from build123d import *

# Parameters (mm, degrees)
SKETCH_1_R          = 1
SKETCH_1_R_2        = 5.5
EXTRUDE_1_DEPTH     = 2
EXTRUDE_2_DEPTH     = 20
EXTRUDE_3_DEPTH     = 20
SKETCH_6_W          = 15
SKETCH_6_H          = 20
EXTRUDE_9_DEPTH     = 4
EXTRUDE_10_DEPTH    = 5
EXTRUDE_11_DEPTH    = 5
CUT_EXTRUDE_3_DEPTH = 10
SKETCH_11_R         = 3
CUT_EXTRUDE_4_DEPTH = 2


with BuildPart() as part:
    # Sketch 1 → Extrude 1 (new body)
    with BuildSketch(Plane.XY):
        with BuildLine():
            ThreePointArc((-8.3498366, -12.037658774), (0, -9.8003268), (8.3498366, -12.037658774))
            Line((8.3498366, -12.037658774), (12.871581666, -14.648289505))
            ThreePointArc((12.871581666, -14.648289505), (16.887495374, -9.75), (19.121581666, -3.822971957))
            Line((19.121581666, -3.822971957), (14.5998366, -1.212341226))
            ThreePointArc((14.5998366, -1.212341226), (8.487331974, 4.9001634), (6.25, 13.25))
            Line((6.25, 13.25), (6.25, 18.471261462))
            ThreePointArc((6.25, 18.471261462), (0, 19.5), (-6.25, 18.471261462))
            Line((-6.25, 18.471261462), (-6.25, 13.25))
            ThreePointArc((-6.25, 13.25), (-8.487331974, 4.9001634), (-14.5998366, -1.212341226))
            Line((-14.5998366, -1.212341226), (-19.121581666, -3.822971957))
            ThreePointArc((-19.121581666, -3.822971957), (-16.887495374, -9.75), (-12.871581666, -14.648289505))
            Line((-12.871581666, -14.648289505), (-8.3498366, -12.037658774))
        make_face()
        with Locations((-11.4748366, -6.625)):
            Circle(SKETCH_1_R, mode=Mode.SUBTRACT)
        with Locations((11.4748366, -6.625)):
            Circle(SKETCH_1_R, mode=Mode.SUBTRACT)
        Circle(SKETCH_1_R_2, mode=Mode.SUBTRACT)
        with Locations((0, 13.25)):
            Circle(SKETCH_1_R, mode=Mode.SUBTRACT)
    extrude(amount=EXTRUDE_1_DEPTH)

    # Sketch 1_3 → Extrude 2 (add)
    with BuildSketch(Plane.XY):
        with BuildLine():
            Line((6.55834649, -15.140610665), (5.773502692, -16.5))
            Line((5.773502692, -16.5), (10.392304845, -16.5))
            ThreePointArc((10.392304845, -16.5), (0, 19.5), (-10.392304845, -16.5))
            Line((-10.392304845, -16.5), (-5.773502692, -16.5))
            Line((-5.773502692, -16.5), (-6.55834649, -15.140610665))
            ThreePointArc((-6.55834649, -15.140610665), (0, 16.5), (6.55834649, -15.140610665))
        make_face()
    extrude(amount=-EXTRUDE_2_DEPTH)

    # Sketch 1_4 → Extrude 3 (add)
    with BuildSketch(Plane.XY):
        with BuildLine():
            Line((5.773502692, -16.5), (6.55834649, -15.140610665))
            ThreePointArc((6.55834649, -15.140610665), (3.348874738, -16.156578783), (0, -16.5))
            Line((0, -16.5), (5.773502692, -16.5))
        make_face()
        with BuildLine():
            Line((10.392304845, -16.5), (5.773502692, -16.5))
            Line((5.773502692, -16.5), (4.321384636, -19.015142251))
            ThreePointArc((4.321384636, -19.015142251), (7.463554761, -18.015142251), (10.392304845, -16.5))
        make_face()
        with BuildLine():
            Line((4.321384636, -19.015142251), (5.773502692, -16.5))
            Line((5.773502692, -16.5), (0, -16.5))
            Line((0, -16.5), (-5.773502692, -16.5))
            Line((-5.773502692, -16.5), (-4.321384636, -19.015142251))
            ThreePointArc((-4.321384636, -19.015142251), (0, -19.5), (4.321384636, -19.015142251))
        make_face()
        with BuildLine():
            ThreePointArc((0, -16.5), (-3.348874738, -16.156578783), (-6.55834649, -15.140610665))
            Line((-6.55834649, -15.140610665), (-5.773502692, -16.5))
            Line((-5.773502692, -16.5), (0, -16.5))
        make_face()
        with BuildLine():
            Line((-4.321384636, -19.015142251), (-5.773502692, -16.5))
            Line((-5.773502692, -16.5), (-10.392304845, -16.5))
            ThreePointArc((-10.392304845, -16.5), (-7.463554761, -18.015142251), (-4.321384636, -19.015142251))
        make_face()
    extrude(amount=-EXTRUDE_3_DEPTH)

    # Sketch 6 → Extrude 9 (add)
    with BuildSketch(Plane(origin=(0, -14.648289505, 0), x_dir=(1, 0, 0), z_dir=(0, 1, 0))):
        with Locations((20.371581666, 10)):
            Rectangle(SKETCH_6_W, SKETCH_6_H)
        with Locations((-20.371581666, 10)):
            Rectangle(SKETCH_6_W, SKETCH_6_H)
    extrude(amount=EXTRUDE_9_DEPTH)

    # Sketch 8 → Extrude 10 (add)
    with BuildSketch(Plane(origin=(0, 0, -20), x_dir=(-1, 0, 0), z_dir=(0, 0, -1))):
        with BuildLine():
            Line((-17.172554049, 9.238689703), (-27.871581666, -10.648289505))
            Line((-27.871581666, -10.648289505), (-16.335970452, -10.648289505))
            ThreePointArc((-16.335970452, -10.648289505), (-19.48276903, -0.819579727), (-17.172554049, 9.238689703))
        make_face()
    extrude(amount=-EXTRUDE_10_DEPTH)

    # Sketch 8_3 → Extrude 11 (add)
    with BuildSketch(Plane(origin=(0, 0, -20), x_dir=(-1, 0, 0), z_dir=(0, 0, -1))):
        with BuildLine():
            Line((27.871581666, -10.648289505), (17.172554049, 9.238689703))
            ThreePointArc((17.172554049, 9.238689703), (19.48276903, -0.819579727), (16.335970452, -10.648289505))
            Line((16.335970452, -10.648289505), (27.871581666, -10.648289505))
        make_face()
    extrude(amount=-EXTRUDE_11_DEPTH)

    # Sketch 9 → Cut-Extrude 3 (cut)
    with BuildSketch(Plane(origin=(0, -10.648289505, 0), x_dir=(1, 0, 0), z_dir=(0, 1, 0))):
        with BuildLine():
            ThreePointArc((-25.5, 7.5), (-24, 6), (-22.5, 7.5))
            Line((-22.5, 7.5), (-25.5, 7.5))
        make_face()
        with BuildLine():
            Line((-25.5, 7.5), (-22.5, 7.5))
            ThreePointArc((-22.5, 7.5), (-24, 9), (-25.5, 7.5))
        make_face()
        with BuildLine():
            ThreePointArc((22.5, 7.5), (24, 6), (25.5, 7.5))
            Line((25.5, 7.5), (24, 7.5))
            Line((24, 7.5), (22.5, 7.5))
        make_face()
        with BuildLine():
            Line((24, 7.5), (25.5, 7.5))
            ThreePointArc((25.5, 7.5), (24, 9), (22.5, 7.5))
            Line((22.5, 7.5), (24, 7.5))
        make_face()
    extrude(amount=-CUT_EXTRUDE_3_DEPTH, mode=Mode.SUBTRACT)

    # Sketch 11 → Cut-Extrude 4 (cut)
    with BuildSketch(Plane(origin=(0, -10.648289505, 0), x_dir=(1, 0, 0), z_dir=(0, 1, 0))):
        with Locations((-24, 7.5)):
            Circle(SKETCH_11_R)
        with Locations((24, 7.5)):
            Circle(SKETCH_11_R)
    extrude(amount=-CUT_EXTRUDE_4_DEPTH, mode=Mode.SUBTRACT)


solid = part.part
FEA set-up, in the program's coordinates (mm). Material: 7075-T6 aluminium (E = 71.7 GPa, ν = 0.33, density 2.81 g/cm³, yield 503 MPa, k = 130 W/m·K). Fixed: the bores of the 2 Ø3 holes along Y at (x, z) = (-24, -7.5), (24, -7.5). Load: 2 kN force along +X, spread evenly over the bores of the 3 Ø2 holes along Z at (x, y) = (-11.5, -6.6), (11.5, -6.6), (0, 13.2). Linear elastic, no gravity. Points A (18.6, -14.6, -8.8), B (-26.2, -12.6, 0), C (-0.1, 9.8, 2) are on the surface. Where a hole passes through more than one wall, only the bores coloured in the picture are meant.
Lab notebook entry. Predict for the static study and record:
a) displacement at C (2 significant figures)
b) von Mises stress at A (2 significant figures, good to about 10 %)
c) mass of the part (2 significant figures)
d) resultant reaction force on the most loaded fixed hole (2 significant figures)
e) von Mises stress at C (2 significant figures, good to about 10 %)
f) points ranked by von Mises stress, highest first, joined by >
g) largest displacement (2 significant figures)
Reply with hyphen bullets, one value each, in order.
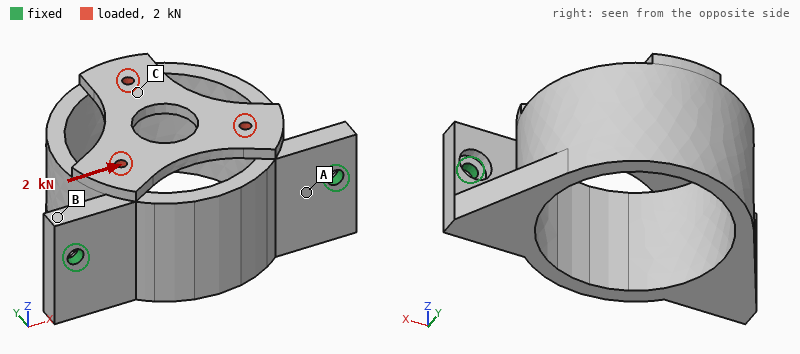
- 45 µm
- 21 MPa
- 30 g
- 1.2 kN
- 51 MPa
- C > A > B
- 48 µm
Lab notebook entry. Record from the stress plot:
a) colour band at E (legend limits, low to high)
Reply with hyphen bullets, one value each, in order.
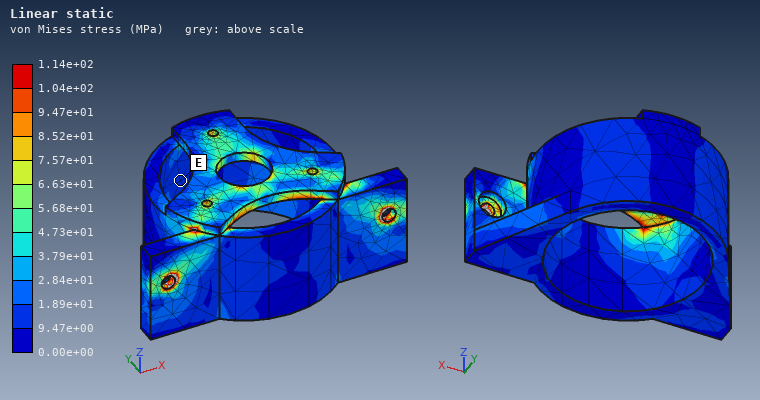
- 9.47e+00 to 1.89e+01 MPa
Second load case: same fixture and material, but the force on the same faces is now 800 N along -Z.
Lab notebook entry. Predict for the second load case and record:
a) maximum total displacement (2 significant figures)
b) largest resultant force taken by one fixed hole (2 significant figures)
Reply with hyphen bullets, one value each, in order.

- 0.37 mm
- 400 N
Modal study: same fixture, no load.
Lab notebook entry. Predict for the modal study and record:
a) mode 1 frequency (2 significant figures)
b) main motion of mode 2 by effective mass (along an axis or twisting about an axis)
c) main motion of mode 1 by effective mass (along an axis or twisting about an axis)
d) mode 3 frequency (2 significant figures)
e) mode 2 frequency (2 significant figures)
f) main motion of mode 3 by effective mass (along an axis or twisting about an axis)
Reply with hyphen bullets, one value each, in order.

- 1700 Hz
- along X
- along Z
- 6900 Hz
- 5800 Hz
- along Y
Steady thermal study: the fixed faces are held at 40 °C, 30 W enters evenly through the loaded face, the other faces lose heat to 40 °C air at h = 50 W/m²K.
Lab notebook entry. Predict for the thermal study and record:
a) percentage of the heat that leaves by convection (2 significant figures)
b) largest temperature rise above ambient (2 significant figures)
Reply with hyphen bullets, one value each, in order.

- 27 %
- 50 K
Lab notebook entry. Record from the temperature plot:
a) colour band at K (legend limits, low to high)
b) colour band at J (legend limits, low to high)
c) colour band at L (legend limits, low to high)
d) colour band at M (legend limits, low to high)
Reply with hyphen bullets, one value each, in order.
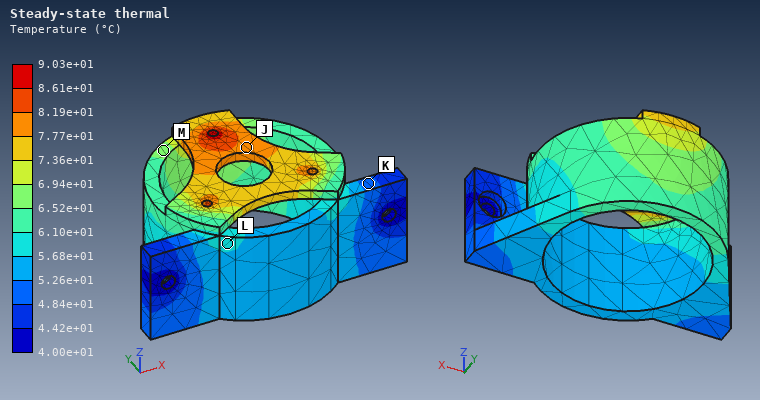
- 4.84e+01 to 5.26e+01 °C
- 7.77e+01 to 8.19e+01 °C
- 5.68e+01 to 6.10e+01 °C
- 6.52e+01 to 6.94e+01 °C
